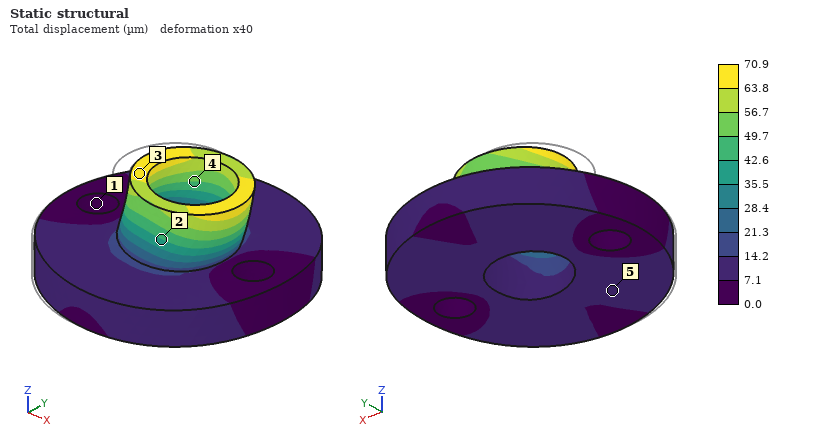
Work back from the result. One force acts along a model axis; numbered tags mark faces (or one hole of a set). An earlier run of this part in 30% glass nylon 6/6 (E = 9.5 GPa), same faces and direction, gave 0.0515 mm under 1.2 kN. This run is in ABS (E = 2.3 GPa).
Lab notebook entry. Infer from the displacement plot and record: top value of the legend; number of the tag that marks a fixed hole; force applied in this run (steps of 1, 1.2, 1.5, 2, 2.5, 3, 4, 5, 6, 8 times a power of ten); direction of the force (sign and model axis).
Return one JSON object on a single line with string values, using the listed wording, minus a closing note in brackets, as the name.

{"top value of the legend": "70.9 µm", "number of the tag that marks a fixed hole": "1", "force applied in this run": "400 N", "direction of the force": "+X"}
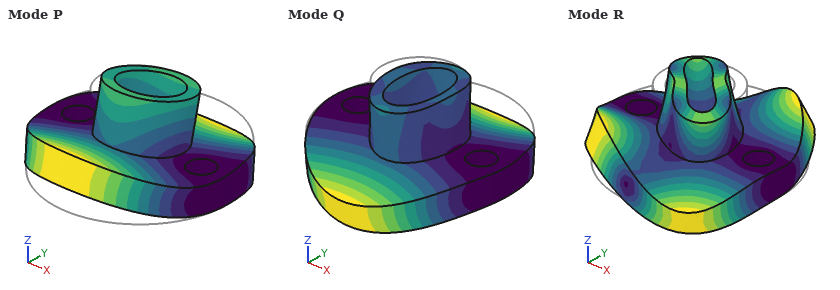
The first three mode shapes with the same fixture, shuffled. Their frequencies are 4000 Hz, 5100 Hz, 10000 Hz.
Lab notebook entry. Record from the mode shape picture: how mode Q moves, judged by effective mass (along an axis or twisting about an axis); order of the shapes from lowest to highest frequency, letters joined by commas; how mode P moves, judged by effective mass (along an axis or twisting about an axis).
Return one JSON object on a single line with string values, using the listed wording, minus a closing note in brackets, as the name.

{"how mode Q moves, judged by effective mass": "along Z", "order of the shapes from lowest to highest frequency, letters joined by commas": "P, Q, R", "how mode P moves, judged by effective mass": "twisting about X"}
